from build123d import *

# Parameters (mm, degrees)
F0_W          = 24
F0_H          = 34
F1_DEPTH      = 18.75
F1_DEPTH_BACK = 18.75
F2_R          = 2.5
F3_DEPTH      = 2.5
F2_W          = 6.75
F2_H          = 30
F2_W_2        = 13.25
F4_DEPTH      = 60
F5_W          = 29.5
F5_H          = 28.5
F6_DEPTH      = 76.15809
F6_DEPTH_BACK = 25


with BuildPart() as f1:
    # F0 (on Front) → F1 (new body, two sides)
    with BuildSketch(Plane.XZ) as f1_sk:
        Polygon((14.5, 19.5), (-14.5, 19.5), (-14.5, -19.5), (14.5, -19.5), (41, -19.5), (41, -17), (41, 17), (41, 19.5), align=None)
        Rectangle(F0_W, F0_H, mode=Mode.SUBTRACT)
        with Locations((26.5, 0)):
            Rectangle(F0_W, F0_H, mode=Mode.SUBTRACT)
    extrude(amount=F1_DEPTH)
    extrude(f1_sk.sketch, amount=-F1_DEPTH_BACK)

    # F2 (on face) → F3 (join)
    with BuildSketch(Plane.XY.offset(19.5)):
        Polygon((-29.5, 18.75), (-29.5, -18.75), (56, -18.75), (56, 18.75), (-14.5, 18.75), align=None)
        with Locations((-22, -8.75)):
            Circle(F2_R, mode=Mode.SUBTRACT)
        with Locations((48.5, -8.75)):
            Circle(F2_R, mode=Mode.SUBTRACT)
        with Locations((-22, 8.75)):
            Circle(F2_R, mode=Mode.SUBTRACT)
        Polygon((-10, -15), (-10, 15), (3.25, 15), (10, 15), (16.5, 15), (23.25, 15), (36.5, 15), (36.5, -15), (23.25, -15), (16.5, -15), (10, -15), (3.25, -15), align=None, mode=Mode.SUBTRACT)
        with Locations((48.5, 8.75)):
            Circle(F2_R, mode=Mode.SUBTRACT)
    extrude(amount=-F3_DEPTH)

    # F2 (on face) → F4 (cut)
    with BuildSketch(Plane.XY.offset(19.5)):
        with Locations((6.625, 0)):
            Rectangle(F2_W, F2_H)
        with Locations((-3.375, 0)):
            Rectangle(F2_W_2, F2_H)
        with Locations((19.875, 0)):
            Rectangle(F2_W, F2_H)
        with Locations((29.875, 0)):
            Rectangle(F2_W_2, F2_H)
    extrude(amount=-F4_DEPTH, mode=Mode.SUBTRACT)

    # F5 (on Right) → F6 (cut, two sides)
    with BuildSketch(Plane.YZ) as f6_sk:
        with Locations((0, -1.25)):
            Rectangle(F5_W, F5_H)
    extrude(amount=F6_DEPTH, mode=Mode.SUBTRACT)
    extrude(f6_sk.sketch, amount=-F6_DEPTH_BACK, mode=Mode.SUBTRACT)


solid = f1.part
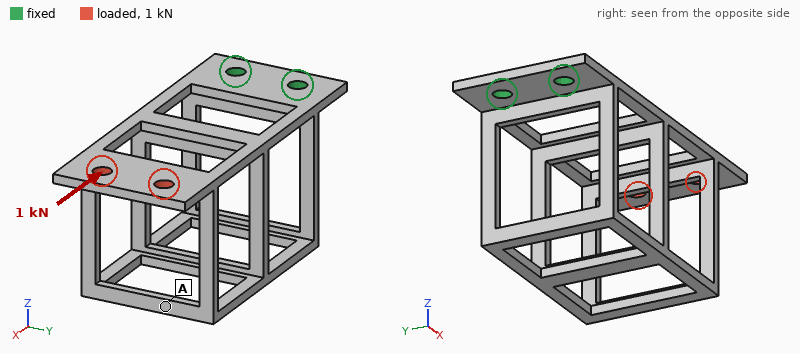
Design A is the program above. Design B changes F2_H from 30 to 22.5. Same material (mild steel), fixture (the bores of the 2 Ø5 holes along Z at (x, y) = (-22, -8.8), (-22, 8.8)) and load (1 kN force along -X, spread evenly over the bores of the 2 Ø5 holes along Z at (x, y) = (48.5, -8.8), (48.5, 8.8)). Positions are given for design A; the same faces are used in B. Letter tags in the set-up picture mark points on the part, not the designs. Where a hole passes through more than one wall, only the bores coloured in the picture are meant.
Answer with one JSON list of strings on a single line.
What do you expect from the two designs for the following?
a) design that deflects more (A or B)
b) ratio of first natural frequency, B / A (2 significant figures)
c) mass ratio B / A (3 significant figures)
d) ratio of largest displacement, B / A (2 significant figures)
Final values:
["A", "1.1", "1.15", "0.52"]
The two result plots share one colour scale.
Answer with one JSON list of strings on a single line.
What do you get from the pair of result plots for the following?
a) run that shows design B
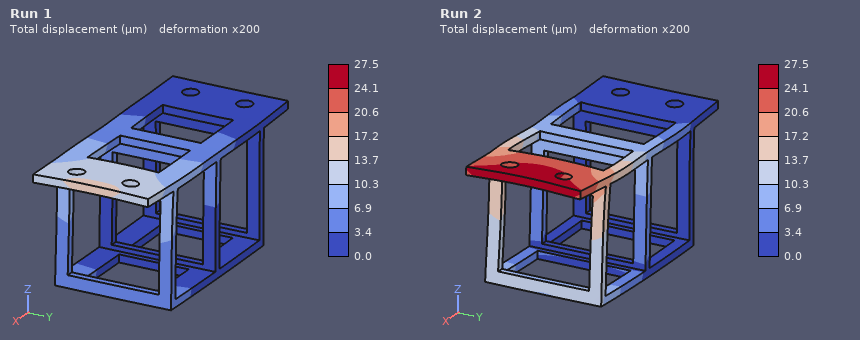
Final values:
["Run 1"]
